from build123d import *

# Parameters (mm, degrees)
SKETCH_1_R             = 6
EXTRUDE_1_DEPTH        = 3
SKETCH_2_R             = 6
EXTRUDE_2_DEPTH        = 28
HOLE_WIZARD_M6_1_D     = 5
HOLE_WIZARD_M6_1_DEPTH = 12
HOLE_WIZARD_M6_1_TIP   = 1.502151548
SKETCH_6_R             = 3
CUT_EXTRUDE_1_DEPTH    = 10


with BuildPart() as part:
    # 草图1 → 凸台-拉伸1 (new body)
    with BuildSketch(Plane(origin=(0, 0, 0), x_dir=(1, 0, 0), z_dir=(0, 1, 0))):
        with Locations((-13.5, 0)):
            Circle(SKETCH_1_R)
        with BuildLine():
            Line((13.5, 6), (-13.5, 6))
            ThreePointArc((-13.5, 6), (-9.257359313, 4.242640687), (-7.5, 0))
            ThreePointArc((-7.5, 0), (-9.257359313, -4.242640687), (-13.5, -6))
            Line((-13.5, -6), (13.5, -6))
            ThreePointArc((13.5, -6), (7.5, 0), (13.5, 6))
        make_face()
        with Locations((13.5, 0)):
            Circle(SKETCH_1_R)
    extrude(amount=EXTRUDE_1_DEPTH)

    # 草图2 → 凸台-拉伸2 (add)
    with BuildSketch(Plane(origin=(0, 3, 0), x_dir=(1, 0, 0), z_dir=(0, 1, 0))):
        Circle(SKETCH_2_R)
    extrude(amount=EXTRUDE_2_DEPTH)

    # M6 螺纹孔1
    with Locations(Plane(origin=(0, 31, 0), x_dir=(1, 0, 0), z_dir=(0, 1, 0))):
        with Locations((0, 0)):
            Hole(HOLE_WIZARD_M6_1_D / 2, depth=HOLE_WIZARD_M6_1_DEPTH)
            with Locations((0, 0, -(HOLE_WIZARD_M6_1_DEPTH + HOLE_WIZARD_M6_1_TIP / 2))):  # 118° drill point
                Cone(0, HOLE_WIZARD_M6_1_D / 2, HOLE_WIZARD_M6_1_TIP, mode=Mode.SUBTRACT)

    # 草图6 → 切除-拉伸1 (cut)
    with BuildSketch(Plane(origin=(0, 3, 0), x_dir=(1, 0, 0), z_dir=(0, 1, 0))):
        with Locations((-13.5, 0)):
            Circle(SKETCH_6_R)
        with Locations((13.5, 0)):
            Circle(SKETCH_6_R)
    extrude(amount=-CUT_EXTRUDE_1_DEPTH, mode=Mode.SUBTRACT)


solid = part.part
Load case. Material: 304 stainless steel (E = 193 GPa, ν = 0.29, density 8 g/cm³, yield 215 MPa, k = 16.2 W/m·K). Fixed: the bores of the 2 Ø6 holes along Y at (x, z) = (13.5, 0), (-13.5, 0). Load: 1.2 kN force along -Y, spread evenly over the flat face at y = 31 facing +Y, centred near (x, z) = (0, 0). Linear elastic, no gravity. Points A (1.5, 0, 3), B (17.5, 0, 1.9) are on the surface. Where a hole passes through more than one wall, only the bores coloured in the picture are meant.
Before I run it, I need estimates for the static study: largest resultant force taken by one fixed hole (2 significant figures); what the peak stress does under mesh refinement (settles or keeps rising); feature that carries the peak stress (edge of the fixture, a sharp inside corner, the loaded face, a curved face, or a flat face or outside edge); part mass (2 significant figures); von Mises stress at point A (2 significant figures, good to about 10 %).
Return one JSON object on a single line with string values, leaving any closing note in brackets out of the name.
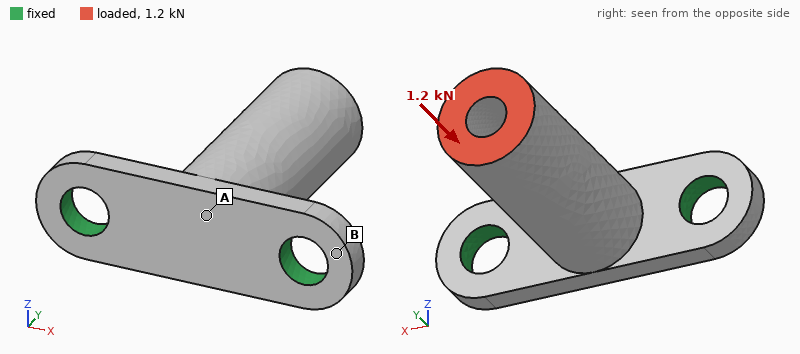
{"largest resultant force taken by one fixed hole": "640 N", "what the peak stress does under mesh refinement": "keeps rising", "feature that carries the peak stress": "edge of the fixture", "part mass": "33 g", "von Mises stress at point A": "31 MPa"}
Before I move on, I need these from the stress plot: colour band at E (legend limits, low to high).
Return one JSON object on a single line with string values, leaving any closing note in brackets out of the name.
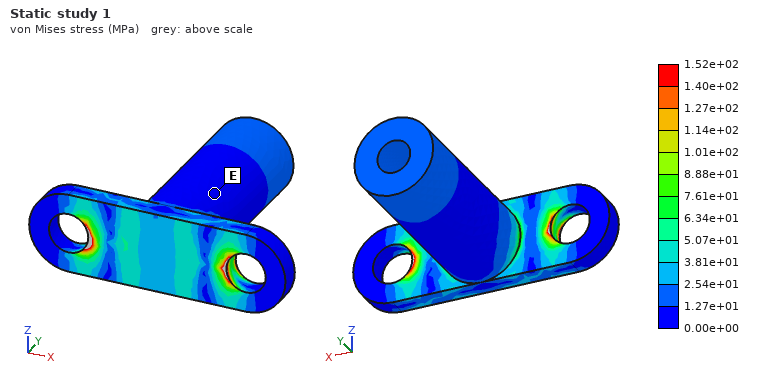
{"colour band at E": "0.00e+00 to 1.27e+01 MPa"}
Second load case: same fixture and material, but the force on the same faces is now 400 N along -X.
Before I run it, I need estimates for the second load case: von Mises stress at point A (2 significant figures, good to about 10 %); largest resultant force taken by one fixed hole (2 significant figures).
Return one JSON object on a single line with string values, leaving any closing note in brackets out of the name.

{"von Mises stress at point A": "27 MPa", "largest resultant force taken by one fixed hole": "720 N"}
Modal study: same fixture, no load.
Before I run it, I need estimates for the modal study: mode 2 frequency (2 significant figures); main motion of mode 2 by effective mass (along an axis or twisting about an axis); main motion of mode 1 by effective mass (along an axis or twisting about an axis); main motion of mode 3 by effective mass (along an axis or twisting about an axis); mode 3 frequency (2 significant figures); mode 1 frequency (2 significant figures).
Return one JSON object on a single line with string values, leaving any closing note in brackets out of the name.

{"mode 2 frequency": "6000 Hz", "main motion of mode 2 by effective mass": "along X", "main motion of mode 1 by effective mass": "along Z", "main motion of mode 3 by effective mass": "along Y", "mode 3 frequency": "13 kHz", "mode 1 frequency": "3000 Hz"}
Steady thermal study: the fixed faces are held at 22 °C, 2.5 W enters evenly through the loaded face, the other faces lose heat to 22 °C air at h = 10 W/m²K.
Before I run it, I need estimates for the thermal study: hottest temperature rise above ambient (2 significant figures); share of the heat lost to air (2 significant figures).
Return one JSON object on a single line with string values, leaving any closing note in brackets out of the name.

{"hottest temperature rise above ambient": "52 K", "share of the heat lost to air": "19 %"}
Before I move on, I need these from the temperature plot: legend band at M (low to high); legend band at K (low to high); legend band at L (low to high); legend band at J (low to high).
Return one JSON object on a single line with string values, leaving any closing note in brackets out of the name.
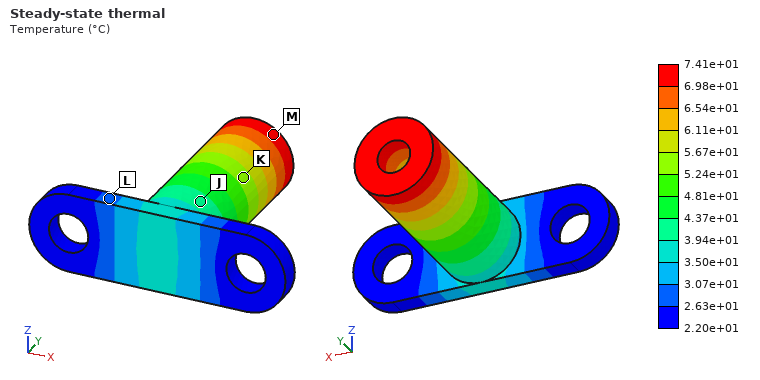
{"legend band at M": "6.98e+01 to 7.41e+01 °C", "legend band at K": "5.24e+01 to 5.67e+01 °C", "legend band at L": "2.63e+01 to 3.07e+01 °C", "legend band at J": "3.94e+01 to 4.37e+01 °C"}
